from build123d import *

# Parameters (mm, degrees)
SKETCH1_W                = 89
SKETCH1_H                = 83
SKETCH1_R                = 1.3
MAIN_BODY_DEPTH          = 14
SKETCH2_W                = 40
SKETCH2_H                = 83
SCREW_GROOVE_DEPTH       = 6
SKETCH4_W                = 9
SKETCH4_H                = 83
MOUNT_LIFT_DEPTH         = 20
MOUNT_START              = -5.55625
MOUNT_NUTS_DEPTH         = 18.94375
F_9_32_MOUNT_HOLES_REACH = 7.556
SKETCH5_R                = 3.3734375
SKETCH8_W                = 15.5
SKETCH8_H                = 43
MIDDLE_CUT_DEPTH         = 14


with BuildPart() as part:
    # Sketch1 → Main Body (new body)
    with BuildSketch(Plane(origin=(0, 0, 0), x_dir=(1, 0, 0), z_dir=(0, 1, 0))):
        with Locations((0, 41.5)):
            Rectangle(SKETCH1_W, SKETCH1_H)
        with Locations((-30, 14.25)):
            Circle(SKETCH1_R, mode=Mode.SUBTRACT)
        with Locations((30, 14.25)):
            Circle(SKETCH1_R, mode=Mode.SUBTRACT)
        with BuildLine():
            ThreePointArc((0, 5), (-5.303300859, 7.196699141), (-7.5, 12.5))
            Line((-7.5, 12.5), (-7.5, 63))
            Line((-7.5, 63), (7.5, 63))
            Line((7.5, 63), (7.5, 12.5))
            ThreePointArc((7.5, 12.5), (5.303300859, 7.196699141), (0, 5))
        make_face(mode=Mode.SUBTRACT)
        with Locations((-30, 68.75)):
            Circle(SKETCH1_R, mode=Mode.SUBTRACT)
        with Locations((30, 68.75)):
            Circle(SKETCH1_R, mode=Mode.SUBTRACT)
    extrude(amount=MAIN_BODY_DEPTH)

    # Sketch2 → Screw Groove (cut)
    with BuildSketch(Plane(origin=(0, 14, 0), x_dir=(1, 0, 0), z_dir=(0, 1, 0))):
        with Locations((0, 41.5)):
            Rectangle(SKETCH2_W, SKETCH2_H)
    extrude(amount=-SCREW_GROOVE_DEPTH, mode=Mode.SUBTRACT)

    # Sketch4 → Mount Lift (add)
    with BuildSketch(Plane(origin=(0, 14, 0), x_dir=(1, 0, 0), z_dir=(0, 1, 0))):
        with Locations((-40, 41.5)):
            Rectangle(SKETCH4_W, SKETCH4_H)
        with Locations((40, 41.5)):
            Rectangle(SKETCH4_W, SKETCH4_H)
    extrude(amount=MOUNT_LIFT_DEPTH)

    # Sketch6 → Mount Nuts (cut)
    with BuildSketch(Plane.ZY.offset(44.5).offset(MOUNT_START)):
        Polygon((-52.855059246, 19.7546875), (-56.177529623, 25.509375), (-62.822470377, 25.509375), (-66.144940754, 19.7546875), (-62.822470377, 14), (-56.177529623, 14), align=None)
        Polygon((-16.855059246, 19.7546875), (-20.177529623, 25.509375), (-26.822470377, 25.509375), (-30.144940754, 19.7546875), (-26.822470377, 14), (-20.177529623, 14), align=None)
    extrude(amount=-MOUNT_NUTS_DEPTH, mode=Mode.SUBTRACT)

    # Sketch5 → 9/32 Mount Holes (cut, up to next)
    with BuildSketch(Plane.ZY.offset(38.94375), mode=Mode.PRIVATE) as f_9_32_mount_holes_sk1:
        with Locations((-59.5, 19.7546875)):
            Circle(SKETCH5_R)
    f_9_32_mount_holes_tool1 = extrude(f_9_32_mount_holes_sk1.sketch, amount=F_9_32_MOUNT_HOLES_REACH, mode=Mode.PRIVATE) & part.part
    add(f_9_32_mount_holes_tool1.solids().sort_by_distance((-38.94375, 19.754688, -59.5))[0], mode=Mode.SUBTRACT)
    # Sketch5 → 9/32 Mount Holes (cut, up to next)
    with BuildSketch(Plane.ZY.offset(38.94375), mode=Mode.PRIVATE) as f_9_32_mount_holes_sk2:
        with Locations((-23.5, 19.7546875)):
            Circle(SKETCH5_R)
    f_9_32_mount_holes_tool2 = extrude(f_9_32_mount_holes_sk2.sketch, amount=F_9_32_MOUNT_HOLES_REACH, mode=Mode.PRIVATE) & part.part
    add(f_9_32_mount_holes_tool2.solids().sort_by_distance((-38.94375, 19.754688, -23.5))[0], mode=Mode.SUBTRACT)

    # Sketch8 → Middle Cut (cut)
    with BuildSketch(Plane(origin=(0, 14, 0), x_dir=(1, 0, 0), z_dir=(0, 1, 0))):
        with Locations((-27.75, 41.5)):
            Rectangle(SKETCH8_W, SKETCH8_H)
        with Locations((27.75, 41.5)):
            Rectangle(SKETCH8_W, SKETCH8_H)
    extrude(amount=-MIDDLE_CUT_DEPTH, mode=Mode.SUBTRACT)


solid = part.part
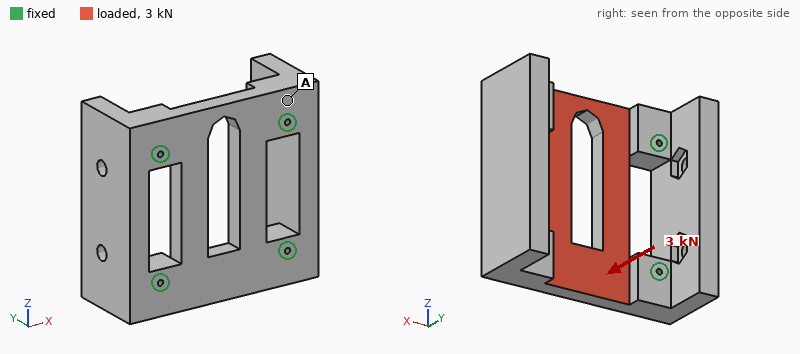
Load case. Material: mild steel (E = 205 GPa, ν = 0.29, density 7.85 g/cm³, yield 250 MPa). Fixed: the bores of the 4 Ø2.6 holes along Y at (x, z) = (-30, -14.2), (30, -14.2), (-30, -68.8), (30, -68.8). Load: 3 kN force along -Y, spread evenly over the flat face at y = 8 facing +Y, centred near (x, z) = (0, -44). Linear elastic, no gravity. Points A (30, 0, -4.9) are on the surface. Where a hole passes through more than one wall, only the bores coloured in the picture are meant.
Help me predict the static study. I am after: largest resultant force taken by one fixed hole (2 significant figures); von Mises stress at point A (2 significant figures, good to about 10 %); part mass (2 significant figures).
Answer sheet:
880 N
6.0 MPa
680 g
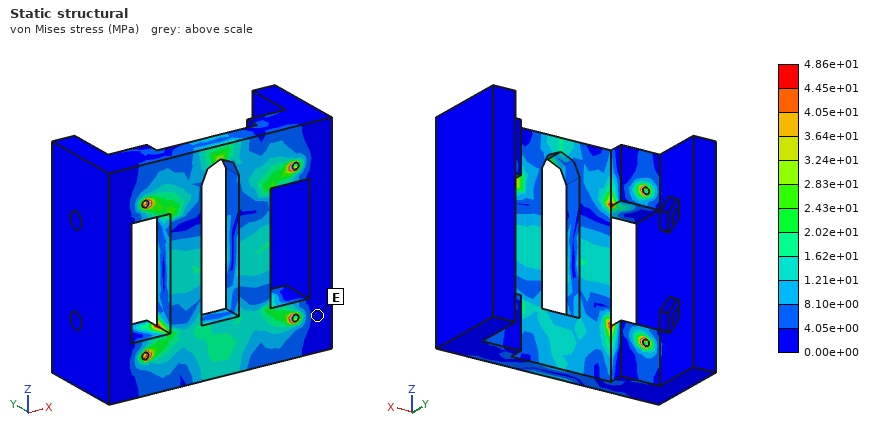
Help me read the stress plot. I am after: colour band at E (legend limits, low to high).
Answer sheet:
0.00e+00 to 4.05e+00 MPa
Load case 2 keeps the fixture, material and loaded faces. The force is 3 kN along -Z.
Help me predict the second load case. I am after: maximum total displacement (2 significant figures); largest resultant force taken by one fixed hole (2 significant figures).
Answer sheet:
2.9 µm
810 N
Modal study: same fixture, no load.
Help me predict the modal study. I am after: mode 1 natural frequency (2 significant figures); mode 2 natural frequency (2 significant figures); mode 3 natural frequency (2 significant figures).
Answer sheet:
6100 Hz
6300 Hz
8900 Hz
